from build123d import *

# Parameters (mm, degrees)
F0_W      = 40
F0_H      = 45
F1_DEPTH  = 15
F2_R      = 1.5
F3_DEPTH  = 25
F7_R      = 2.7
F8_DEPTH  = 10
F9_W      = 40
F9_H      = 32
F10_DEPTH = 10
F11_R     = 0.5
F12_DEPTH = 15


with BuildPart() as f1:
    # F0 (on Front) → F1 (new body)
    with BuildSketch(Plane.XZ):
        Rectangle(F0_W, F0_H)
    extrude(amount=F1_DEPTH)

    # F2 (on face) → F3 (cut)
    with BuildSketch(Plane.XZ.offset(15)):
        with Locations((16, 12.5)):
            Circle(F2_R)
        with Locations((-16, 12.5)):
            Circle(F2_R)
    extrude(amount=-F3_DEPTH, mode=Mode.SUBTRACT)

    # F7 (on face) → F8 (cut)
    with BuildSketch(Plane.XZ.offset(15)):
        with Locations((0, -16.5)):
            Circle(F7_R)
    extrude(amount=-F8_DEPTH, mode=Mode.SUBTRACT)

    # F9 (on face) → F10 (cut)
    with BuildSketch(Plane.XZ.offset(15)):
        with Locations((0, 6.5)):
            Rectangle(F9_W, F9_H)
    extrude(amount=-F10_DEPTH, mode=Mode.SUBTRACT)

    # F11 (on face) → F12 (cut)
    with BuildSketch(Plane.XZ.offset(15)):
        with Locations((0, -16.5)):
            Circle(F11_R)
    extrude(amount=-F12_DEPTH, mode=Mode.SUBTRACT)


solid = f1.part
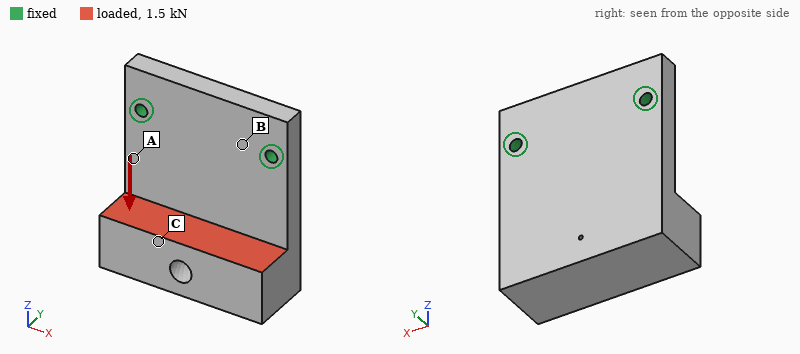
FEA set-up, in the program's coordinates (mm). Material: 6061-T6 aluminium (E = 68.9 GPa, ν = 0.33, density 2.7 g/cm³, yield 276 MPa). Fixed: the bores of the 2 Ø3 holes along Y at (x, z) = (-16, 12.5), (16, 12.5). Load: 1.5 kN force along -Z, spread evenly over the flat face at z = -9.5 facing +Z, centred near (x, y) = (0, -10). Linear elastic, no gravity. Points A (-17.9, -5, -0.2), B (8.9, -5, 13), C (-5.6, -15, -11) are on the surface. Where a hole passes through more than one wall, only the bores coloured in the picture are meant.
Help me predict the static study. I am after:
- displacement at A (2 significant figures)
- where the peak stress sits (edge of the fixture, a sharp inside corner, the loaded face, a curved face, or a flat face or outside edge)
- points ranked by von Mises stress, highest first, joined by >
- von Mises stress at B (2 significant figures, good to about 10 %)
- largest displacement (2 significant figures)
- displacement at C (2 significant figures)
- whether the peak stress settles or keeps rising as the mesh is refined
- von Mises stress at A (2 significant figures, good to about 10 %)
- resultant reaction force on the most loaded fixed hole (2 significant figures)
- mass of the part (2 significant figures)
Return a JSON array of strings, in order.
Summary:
["0.044 mm", "edge of the fixture", "A > B > C", "38 MPa", "0.28 mm", "0.18 mm", "keeps rising", "79 MPa", "760 N", "38 g"]
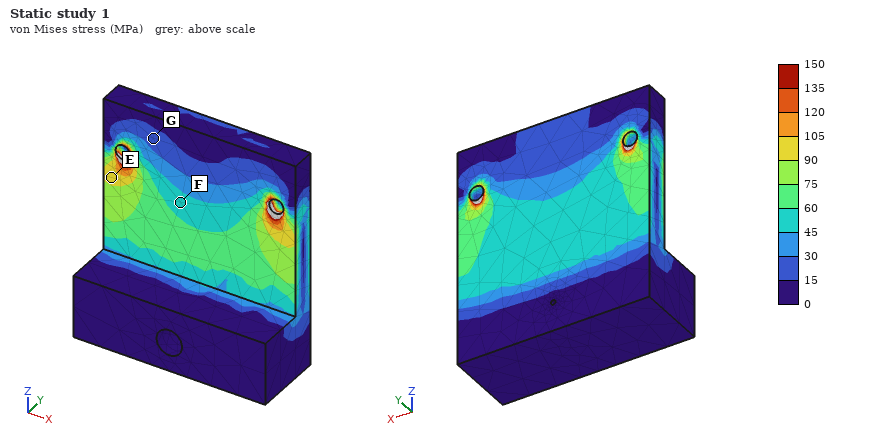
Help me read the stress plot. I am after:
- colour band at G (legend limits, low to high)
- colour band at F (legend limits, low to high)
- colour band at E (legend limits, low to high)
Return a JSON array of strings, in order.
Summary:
["15 to 30 MPa", "45 to 60 MPa", "90 to 105 MPa"]
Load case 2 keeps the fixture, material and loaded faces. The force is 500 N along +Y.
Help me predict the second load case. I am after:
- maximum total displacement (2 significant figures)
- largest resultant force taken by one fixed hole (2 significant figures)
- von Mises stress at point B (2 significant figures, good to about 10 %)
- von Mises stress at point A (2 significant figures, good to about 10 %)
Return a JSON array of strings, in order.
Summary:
["0.17 mm", "250 N", "29 MPa", "32 MPa"]
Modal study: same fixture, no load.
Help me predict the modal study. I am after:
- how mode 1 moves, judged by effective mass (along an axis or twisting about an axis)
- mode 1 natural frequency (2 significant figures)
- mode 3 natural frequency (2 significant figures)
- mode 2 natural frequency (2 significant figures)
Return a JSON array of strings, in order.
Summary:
["along Y", "1700 Hz", "10 kHz", "5000 Hz"]
